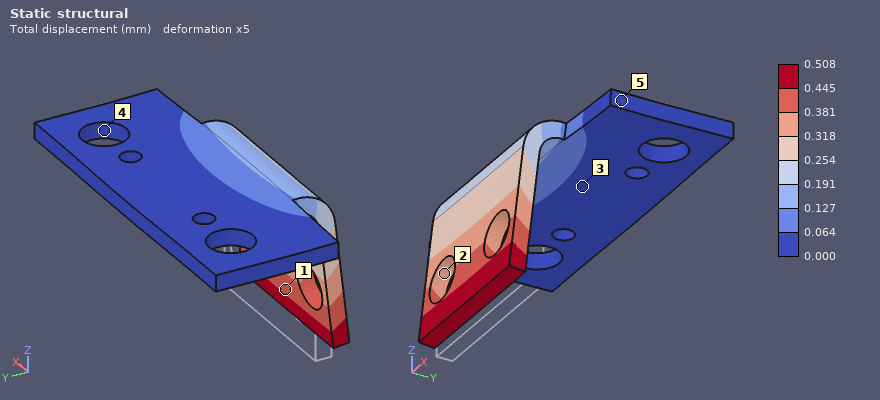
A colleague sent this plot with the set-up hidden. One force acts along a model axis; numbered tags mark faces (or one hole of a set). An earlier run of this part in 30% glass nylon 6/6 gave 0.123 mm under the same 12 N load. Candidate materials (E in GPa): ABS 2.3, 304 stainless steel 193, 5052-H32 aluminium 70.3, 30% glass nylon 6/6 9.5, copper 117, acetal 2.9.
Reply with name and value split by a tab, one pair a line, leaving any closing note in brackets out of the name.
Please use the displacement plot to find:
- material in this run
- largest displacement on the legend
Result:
material in this run	ABS
largest displacement on the legend	0.508 mm
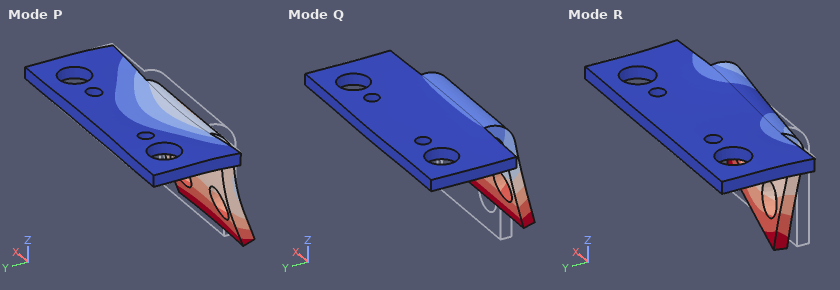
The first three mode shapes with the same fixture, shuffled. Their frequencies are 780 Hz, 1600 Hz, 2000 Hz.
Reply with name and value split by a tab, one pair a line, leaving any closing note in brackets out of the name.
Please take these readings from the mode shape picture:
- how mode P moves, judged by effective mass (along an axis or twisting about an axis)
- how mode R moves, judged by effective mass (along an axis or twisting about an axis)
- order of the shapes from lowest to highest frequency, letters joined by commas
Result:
how mode P moves, judged by effective mass	along Z
how mode R moves, judged by effective mass	along X
order of the shapes from lowest to highest frequency, letters joined by commas	Q, R, P
